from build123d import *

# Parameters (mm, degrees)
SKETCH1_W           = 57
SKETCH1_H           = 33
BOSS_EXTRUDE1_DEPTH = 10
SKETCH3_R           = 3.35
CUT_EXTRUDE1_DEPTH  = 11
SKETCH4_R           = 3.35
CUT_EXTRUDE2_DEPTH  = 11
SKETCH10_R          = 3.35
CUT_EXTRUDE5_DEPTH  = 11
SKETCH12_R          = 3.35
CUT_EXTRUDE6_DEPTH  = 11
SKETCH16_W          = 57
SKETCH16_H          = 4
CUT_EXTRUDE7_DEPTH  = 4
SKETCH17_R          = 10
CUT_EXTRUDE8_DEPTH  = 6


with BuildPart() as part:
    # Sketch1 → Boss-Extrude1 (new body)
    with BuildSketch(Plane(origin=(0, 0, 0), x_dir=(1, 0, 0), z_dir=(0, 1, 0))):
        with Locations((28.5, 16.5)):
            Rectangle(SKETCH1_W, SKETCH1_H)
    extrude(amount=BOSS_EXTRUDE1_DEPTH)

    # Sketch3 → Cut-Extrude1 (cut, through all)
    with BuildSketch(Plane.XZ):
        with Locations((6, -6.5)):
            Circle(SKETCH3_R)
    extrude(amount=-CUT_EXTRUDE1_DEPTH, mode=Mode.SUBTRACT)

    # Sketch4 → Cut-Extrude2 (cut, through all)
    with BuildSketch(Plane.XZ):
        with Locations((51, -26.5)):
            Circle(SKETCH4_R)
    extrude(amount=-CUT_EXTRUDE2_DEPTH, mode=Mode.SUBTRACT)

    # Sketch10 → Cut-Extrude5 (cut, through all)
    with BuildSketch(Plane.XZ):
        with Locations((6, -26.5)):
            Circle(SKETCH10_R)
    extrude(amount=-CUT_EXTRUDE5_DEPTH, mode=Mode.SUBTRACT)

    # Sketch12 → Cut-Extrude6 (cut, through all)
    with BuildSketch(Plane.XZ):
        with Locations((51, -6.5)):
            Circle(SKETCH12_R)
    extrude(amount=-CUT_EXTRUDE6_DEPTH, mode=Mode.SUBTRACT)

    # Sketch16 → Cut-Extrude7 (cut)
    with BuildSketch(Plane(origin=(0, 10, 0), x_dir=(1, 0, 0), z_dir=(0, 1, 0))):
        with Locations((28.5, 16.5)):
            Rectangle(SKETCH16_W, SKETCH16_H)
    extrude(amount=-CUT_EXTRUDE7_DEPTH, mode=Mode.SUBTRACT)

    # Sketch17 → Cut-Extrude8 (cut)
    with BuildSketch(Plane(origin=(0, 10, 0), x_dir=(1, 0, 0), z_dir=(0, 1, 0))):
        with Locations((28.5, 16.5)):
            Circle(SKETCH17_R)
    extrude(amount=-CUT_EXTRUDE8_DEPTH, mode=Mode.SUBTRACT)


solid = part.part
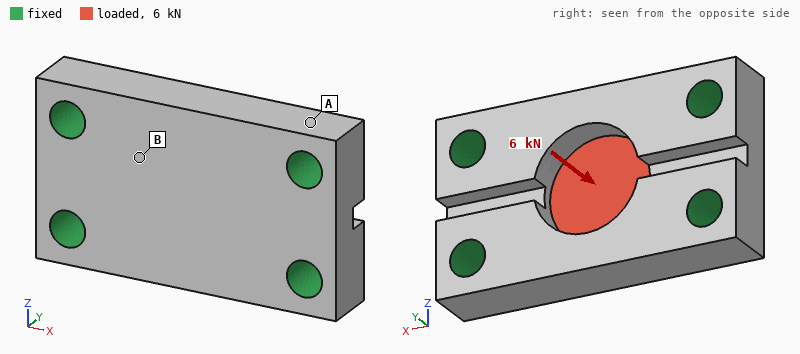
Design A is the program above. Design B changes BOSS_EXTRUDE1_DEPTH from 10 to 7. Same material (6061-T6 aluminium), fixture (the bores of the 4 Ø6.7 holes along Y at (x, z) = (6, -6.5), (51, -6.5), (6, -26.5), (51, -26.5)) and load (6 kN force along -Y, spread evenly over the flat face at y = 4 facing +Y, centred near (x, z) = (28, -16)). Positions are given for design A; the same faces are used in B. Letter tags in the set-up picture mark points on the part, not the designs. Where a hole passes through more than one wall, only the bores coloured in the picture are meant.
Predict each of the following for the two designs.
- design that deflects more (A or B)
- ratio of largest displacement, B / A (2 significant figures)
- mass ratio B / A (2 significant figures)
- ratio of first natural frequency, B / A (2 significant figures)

B
1.7
0.74
0.78
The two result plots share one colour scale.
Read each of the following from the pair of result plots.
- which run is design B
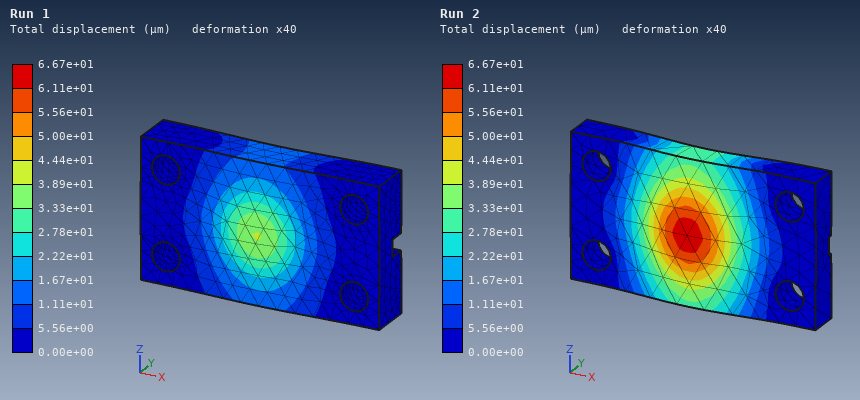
Run 2
